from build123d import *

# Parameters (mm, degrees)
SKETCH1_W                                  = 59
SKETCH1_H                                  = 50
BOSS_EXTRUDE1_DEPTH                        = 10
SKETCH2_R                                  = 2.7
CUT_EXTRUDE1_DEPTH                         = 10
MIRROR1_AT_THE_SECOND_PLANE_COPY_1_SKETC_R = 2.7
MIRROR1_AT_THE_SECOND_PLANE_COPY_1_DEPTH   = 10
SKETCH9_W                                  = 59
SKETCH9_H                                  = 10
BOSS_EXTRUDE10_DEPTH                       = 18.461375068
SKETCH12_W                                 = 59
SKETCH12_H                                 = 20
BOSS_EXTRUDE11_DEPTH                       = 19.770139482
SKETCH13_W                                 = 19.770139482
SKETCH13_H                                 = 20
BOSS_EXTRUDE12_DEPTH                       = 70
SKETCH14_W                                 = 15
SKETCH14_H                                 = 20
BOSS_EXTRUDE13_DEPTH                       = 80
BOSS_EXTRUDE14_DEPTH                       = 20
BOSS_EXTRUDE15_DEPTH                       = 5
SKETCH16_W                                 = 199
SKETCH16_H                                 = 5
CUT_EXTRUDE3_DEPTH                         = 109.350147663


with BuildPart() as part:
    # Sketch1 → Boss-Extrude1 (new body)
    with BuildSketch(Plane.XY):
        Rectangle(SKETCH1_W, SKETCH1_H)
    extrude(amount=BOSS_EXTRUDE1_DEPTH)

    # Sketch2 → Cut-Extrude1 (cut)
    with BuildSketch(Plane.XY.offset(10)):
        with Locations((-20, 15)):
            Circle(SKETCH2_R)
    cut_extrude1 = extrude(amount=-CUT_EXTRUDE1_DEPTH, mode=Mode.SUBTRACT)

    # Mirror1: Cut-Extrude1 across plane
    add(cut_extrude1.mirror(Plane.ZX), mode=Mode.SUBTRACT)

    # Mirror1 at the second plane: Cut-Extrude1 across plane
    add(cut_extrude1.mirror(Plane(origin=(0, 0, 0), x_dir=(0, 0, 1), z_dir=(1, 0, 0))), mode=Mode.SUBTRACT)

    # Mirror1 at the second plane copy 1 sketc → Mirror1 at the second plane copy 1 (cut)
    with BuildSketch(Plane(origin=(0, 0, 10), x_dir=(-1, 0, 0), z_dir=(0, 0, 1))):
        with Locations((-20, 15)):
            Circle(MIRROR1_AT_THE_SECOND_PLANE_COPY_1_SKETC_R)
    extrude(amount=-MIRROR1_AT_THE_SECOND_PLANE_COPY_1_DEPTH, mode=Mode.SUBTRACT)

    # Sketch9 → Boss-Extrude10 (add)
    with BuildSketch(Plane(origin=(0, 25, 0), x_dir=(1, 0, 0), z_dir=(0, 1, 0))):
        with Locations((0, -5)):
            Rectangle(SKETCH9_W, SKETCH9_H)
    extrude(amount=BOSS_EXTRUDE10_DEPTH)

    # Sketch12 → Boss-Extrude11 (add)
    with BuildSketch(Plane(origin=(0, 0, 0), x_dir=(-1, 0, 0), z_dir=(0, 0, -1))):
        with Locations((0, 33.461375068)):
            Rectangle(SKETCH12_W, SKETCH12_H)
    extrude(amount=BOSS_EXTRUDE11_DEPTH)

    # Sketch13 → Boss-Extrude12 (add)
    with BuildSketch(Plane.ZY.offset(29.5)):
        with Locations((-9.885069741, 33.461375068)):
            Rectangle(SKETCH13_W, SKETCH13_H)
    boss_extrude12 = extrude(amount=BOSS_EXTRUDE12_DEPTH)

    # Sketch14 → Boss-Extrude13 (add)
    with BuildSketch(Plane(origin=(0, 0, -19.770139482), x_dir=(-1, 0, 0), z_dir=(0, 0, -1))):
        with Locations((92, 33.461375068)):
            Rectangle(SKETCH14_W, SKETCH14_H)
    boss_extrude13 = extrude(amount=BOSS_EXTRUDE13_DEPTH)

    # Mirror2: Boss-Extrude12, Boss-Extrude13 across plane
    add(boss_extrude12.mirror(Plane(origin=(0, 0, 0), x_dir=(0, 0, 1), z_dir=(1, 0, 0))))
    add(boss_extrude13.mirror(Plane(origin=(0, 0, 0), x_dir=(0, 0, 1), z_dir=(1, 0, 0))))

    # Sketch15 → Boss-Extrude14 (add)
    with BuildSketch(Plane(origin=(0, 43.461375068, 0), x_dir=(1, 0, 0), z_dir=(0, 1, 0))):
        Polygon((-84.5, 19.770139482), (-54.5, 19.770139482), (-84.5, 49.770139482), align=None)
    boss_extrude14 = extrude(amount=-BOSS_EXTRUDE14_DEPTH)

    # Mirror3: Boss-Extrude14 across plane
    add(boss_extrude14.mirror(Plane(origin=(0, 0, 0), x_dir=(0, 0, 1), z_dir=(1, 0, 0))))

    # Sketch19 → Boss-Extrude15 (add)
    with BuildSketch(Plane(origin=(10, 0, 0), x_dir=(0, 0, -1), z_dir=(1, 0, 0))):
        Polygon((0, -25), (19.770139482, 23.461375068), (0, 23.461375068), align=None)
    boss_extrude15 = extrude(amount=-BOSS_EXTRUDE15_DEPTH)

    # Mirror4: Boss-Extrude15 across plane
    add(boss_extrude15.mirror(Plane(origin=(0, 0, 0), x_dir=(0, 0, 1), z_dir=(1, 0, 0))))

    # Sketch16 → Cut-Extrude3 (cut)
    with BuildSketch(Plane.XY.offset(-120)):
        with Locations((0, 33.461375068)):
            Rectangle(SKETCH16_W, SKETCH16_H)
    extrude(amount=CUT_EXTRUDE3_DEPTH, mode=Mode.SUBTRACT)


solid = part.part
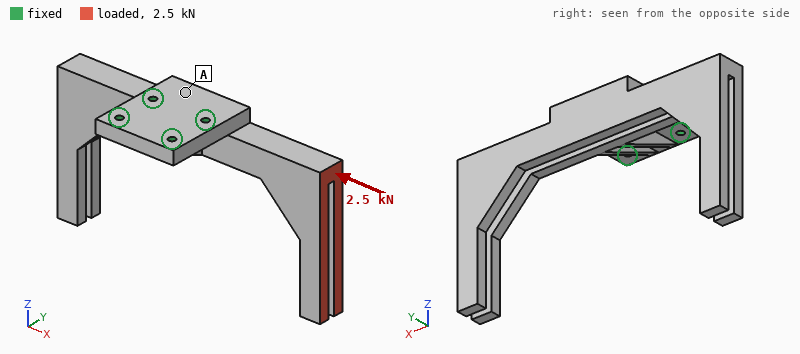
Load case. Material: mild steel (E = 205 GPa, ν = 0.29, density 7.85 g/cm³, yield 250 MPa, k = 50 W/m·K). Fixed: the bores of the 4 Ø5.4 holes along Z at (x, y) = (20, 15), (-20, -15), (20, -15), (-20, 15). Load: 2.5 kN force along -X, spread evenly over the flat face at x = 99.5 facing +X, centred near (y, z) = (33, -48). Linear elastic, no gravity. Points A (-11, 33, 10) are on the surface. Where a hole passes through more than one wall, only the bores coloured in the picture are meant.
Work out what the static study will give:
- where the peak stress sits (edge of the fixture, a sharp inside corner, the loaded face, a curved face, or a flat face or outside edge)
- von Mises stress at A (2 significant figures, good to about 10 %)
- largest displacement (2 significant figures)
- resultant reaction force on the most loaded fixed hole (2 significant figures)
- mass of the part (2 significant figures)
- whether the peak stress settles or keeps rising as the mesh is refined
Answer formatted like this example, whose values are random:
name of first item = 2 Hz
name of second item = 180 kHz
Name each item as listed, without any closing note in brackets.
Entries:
where the peak stress sits = edge of the fixture
von Mises stress at A = 14 MPa
largest displacement = 0.32 mm
resultant reaction force on the most loaded fixed hole = 3.7 kN
mass of the part = 1.3 kg
whether the peak stress settles or keeps rising as the mesh is refined = keeps rising
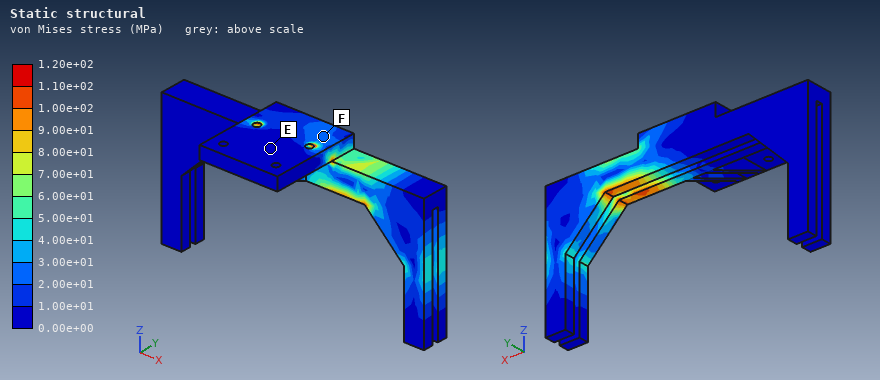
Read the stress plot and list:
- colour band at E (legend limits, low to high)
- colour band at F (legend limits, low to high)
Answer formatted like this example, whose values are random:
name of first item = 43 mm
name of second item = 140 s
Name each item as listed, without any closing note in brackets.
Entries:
colour band at E = 0.00e+00 to 1.00e+01 MPa
colour band at F = 2.00e+01 to 3.00e+01 MPa
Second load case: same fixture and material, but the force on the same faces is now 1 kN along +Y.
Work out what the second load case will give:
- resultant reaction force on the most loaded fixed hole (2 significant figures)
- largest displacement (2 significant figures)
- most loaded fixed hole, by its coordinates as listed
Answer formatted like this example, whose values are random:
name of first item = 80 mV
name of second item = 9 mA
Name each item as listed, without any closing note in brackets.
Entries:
resultant reaction force on the most loaded fixed hole = 2.6 kN
largest displacement = 0.61 mm
most loaded fixed hole, by its coordinates as listed = (20, 15)
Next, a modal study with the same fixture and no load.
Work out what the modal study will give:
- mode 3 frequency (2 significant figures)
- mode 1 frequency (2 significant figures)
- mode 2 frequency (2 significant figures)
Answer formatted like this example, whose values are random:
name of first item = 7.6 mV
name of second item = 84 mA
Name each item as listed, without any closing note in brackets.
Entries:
mode 3 frequency = 850 Hz
mode 1 frequency = 580 Hz
mode 2 frequency = 590 Hz
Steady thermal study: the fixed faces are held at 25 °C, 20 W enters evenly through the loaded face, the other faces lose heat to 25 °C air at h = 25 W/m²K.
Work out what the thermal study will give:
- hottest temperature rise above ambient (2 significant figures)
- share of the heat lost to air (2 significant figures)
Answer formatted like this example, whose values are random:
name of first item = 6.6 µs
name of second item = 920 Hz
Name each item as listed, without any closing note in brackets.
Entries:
hottest temperature rise above ambient = 54 K
share of the heat lost to air = 67 %
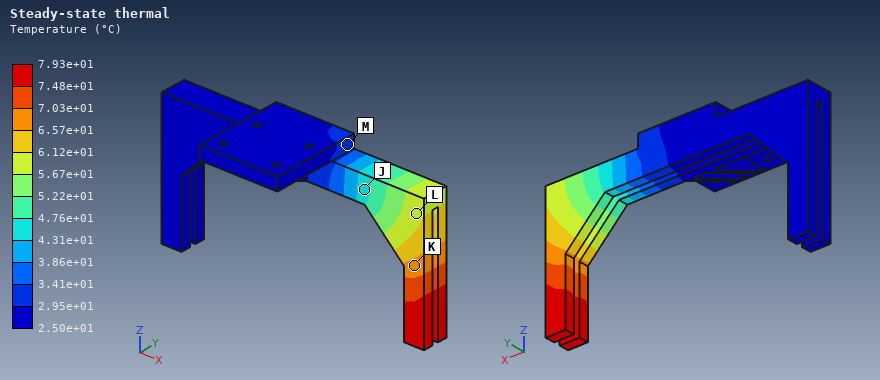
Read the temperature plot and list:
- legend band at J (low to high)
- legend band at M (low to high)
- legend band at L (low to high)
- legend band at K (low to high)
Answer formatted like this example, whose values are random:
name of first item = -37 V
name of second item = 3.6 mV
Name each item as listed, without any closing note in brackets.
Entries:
legend band at J = 4.31e+01 to 4.76e+01 °C
legend band at M = 2.95e+01 to 3.41e+01 °C
legend band at L = 5.67e+01 to 6.12e+01 °C
legend band at K = 6.57e+01 to 7.03e+01 °C
